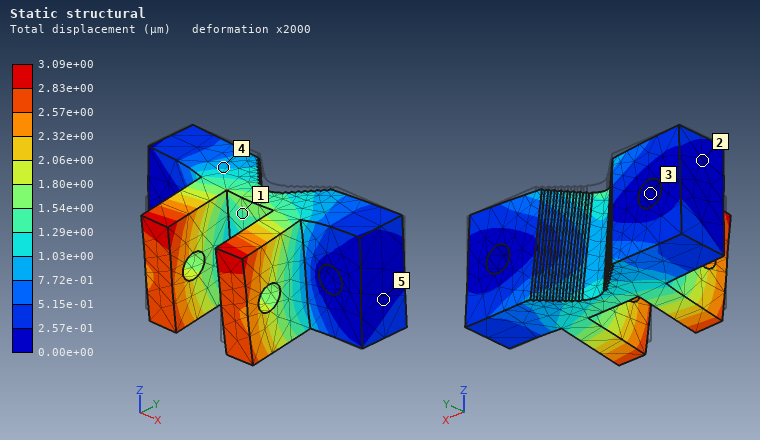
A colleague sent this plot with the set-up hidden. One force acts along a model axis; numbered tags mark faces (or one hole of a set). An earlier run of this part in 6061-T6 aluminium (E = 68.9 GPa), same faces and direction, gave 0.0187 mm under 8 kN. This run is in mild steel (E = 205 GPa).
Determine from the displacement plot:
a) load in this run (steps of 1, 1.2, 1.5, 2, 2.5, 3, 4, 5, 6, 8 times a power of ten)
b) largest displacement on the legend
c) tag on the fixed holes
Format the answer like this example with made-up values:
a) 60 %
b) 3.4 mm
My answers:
a) 4 kN
b) 3.09e+00 µm
c) 3
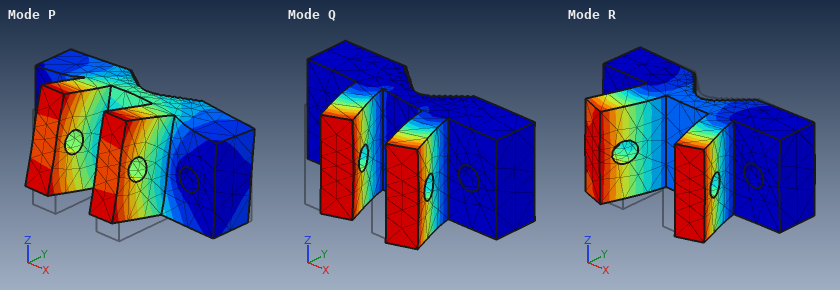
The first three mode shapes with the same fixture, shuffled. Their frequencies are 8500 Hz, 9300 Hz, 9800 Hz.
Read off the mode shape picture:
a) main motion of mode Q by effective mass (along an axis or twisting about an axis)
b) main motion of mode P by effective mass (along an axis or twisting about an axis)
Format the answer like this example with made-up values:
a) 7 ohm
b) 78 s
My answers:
a) along X
b) along Z
